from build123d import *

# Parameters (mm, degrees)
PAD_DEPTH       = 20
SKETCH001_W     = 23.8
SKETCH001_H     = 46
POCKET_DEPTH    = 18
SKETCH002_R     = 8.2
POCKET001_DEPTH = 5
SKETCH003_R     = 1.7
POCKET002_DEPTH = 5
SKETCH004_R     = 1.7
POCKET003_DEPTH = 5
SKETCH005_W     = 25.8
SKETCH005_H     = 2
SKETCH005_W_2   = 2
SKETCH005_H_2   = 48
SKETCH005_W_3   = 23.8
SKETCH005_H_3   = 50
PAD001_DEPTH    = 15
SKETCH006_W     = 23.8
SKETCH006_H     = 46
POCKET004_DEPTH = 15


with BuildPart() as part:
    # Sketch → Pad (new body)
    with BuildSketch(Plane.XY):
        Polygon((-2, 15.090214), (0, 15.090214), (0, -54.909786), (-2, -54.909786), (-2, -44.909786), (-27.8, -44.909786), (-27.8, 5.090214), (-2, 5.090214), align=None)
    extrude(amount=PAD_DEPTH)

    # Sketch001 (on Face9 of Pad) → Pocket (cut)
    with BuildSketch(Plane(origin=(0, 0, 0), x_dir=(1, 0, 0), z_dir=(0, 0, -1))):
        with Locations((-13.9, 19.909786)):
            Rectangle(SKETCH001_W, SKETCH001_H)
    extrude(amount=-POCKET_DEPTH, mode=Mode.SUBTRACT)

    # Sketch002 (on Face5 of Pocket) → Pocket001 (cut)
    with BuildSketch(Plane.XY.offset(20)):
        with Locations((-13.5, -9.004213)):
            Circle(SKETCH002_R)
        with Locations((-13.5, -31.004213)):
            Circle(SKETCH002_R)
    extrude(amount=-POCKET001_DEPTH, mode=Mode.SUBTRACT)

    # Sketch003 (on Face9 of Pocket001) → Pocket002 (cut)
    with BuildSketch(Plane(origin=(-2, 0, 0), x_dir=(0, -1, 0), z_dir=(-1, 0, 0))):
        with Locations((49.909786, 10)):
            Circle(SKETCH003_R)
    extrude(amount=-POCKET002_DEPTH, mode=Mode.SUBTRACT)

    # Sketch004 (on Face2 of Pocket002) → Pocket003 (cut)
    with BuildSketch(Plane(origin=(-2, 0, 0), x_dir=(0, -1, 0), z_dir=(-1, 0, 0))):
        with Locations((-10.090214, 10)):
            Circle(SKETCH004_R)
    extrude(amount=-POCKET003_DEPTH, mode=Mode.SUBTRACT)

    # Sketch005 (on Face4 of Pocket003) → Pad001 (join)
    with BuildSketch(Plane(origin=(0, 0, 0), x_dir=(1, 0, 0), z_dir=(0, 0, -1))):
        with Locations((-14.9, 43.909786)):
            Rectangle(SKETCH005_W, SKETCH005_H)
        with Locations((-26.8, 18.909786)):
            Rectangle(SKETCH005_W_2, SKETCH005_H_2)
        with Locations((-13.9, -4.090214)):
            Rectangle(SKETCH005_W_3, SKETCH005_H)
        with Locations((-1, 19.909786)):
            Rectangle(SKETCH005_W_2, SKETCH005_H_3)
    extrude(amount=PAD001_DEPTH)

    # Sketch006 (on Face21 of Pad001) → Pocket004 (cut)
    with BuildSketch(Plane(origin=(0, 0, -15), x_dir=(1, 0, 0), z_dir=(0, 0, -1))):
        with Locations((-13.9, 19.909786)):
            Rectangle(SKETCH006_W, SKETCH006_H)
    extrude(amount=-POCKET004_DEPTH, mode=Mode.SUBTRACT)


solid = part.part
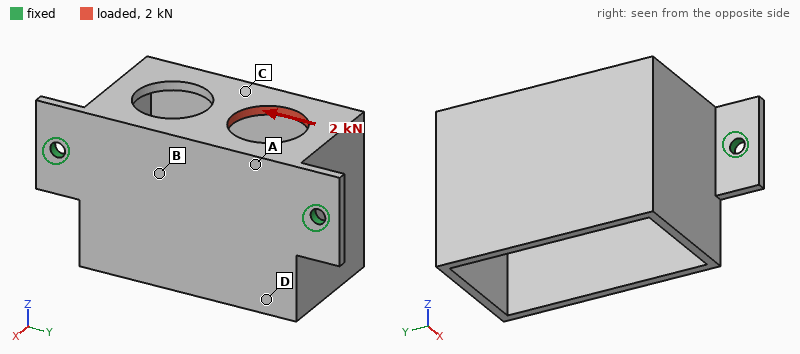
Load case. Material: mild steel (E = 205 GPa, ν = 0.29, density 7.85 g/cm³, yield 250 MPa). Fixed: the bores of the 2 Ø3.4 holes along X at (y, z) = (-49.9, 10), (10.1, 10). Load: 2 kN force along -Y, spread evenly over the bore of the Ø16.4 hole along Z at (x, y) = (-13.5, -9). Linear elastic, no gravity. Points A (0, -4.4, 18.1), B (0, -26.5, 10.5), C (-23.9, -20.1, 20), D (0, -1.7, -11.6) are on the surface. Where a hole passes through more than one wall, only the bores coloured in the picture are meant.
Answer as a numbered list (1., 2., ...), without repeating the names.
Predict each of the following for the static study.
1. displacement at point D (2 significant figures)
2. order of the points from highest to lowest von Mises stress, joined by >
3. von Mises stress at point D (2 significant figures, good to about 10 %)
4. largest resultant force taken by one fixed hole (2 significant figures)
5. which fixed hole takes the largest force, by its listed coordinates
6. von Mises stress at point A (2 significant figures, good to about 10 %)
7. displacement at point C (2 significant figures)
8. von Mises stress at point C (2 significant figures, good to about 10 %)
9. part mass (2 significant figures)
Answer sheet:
1. 13 µm
2. A > C > D > B
3. 24 MPa
4. 1.2 kN
5. (10.1, 10)
6. 54 MPa
7. 26 µm
8. 37 MPa
9. 98 g
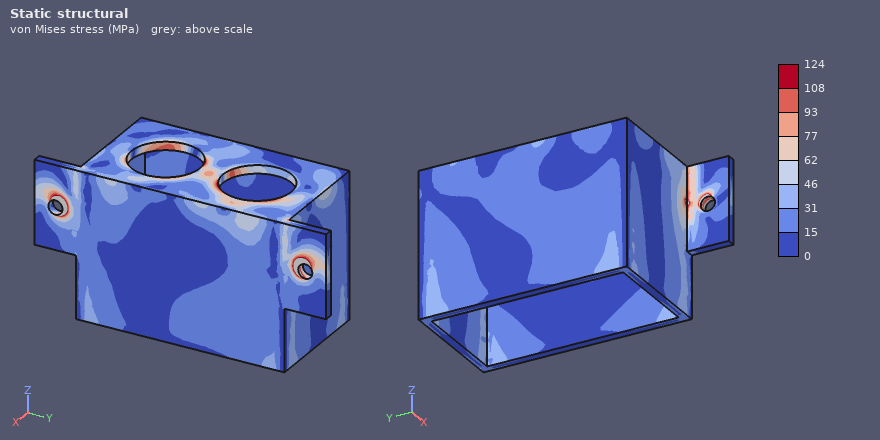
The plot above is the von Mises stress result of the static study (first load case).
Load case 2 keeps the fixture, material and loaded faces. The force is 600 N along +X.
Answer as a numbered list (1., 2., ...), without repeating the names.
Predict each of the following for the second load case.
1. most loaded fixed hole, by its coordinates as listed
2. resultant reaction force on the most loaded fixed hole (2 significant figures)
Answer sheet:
1. (10.1, 10)
2. 440 N
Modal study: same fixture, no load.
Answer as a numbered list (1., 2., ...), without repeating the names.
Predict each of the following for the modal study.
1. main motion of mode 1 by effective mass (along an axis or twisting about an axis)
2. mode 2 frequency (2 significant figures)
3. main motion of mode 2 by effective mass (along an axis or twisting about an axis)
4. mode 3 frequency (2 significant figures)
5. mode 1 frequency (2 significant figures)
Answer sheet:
1. along Z
2. 2100 Hz
3. along Y
4. 3800 Hz
5. 1100 Hz
